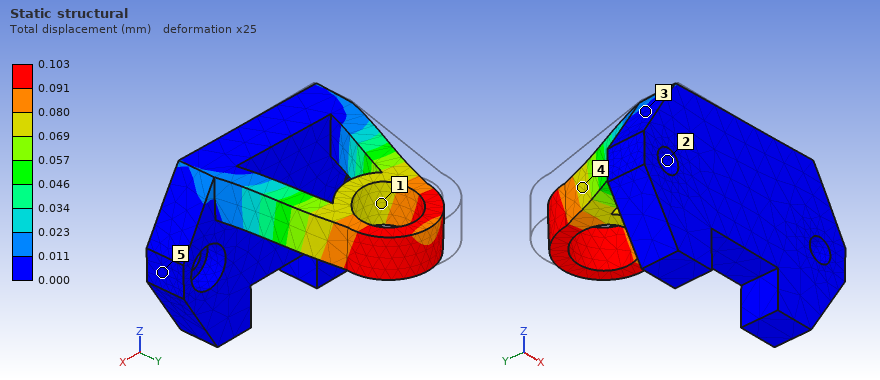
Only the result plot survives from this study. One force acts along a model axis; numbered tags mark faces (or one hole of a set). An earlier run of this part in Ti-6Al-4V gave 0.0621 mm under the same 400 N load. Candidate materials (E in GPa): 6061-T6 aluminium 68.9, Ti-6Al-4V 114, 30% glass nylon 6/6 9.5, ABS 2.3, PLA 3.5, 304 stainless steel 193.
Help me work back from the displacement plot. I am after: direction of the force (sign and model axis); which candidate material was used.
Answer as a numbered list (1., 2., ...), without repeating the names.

1. +X
2. 6061-T6 aluminium
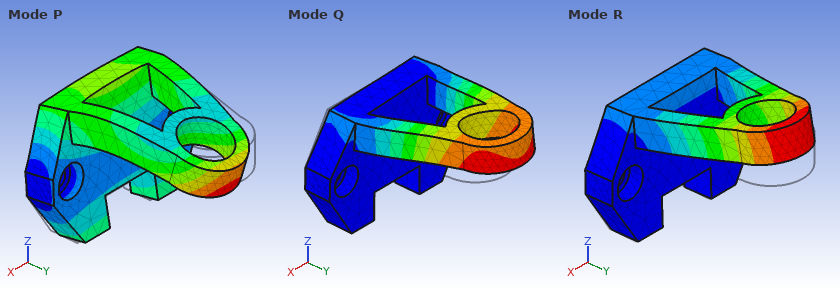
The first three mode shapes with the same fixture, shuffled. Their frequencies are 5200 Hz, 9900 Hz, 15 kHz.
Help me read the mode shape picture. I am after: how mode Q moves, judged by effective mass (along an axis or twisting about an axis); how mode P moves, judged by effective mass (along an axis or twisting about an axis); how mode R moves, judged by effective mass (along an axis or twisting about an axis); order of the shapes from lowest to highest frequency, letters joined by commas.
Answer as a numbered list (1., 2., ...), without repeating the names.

1. along X
2. along Y
3. along Z
4. R, Q, P
